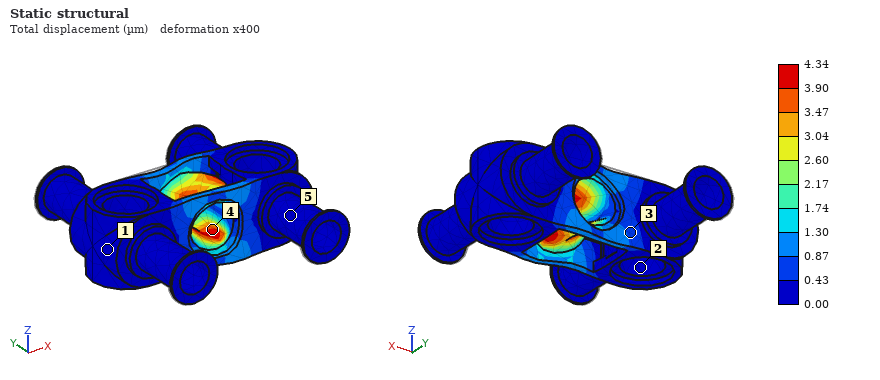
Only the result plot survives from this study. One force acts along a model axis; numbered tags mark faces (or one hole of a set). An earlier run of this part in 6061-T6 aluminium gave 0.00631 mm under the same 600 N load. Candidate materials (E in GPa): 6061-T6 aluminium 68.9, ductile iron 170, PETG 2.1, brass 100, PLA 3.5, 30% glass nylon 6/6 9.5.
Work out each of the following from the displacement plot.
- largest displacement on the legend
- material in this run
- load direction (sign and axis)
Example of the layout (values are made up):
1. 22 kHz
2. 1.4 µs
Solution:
1. 4.34 µm
2. brass
3. +X
